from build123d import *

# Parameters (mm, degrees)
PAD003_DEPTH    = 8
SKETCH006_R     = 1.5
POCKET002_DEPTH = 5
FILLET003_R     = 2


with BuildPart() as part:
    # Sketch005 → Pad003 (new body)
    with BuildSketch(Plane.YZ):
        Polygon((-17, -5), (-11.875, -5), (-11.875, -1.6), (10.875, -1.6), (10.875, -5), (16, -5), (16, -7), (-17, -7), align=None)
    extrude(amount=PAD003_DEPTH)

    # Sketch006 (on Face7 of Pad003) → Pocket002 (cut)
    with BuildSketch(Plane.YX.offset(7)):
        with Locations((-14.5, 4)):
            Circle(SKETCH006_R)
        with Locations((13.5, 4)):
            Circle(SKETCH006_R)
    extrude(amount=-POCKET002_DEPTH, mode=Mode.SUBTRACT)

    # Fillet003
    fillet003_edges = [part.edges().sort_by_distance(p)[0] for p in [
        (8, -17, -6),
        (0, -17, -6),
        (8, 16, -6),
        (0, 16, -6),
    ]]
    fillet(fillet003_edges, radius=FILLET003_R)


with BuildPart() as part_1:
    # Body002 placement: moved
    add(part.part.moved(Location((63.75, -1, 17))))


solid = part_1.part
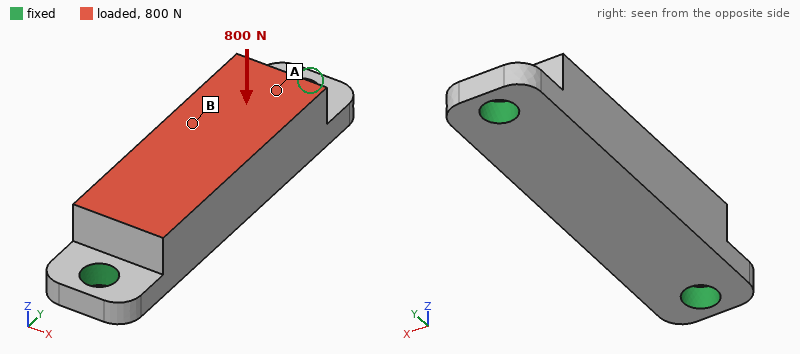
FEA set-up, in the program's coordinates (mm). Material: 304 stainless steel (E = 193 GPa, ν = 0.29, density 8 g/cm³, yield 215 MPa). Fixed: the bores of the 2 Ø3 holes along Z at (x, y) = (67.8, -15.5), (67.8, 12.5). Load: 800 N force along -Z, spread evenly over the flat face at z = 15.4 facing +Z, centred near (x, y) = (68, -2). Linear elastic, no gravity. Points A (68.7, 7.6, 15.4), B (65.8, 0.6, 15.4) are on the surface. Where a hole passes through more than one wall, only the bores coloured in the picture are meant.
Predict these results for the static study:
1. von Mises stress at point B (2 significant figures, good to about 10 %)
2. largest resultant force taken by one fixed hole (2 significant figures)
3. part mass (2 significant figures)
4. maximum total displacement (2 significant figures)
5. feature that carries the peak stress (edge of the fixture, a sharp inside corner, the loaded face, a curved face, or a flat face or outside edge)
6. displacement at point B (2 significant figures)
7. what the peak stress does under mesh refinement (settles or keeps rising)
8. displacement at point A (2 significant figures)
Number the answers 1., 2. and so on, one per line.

1. 47 MPa
2. 560 N
3. 8.9 g
4. 6.7 µm
5. edge of the fixture
6. 6.3 µm
7. keeps rising
8. 3.7 µm
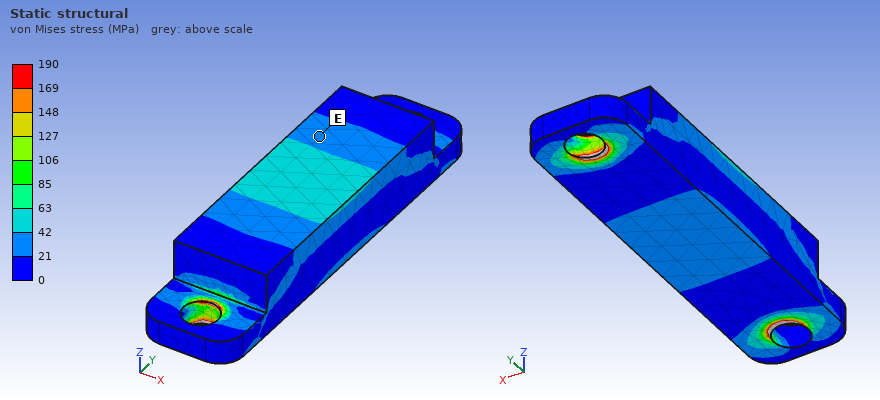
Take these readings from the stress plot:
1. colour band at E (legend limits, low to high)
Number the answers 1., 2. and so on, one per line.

1. 21 to 42 MPa
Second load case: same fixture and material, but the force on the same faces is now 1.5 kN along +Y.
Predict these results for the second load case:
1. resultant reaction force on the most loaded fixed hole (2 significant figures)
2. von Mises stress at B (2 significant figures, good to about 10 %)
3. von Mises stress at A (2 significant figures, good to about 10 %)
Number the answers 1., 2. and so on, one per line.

1. 800 N
2. 14 MPa
3. 20 MPa
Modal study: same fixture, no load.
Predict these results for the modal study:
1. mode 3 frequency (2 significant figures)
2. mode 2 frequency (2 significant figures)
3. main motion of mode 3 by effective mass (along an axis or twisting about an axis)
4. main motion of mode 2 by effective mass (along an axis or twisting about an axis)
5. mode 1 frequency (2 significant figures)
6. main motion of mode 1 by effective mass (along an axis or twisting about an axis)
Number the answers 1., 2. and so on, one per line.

1. 32 kHz
2. 22 kHz
3. along X
4. along Z
5. 19 kHz
6. along X
